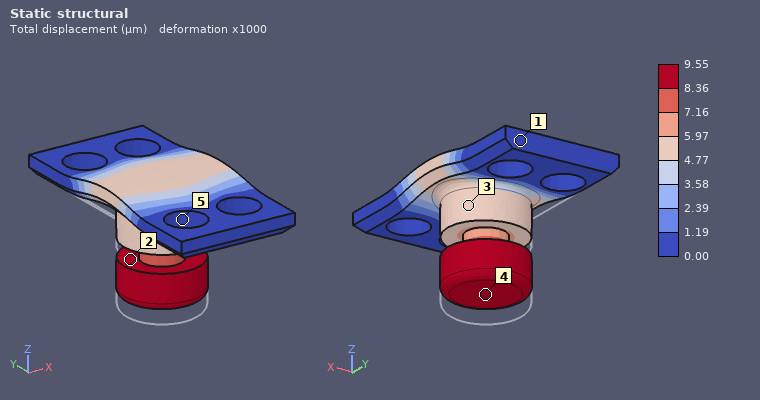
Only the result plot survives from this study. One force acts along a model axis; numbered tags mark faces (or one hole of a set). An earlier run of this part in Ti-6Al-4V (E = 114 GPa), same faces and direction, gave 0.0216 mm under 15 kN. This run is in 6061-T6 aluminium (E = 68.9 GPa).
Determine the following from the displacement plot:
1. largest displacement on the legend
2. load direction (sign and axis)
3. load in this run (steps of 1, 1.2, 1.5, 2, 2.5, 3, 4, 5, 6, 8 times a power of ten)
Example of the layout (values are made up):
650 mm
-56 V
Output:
9.55 µm
+Z
4 kN
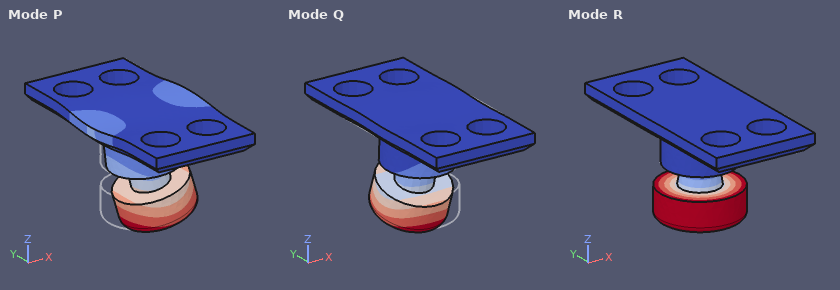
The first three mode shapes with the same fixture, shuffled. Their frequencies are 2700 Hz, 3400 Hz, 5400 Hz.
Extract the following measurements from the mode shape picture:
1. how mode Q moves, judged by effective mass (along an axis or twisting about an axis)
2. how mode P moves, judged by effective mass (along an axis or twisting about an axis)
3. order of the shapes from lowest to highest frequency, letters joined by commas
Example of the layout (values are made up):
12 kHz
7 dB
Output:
along Y
along X
P, Q, R
